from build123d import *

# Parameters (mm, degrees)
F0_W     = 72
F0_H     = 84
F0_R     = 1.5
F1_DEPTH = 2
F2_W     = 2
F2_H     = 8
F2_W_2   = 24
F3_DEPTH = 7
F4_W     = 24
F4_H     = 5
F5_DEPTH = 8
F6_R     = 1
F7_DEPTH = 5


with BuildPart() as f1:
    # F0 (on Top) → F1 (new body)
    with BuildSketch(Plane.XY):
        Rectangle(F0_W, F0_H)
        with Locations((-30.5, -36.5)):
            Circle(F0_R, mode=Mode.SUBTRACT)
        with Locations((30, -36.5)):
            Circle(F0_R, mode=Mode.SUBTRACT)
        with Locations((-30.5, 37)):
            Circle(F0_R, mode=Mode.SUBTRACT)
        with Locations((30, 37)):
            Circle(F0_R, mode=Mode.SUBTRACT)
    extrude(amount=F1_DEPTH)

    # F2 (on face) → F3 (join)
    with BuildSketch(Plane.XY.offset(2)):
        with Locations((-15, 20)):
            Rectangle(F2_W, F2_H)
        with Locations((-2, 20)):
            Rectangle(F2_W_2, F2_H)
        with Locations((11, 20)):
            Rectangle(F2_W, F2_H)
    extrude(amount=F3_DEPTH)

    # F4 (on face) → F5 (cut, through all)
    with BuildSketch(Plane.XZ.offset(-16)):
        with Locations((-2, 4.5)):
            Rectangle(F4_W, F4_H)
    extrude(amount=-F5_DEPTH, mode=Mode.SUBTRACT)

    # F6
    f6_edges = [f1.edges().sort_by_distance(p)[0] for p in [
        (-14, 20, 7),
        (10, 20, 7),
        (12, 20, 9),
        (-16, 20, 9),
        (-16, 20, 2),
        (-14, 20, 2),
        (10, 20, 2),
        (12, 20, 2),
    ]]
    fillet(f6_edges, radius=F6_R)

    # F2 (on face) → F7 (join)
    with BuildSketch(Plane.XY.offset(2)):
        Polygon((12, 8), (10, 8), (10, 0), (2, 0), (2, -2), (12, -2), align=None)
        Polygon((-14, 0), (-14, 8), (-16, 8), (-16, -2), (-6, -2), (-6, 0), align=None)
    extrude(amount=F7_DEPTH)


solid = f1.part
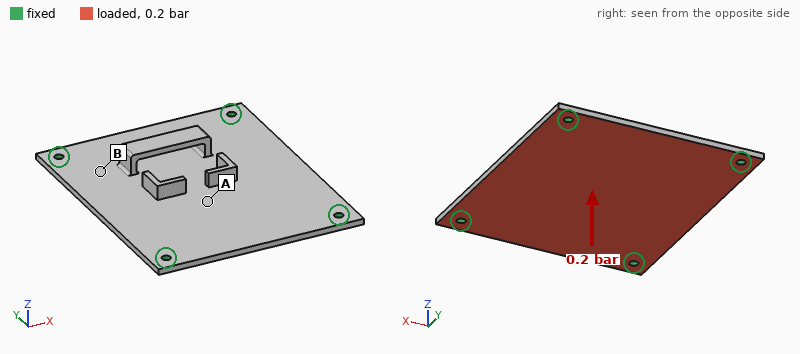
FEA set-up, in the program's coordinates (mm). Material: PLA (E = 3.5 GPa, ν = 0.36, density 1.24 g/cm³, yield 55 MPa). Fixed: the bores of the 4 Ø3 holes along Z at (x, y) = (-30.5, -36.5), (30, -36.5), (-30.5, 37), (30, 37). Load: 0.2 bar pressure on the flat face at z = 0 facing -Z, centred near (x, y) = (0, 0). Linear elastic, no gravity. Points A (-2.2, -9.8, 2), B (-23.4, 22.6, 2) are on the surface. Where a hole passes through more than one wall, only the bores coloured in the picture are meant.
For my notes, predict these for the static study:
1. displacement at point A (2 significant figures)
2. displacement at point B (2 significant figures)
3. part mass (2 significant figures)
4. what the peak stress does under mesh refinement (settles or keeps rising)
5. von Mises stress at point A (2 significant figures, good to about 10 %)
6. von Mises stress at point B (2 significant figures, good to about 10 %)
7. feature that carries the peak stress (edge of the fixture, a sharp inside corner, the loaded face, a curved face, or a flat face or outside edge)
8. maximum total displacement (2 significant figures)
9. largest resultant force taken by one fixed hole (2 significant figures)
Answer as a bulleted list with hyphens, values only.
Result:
- 1.1 mm
- 0.51 mm
- 16 g
- keeps rising
- 7.1 MPa
- 2.9 MPa
- edge of the fixture
- 1.1 mm
- 31 N
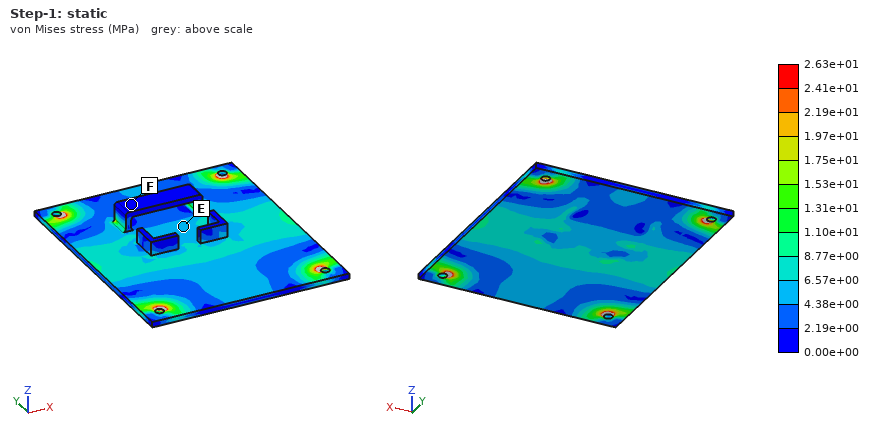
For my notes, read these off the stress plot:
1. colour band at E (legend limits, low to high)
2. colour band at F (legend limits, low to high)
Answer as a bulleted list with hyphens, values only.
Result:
- 4.38e+00 to 6.57e+00 MPa
- 0.00e+00 to 2.19e+00 MPa
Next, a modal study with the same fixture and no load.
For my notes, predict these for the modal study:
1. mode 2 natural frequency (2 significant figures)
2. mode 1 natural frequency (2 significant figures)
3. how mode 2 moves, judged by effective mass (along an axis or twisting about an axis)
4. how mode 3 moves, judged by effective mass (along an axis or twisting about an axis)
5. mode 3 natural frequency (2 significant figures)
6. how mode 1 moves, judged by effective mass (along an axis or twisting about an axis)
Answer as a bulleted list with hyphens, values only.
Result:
- 770 Hz
- 470 Hz
- twisting about Y
- twisting about X
- 970 Hz
- along Z
